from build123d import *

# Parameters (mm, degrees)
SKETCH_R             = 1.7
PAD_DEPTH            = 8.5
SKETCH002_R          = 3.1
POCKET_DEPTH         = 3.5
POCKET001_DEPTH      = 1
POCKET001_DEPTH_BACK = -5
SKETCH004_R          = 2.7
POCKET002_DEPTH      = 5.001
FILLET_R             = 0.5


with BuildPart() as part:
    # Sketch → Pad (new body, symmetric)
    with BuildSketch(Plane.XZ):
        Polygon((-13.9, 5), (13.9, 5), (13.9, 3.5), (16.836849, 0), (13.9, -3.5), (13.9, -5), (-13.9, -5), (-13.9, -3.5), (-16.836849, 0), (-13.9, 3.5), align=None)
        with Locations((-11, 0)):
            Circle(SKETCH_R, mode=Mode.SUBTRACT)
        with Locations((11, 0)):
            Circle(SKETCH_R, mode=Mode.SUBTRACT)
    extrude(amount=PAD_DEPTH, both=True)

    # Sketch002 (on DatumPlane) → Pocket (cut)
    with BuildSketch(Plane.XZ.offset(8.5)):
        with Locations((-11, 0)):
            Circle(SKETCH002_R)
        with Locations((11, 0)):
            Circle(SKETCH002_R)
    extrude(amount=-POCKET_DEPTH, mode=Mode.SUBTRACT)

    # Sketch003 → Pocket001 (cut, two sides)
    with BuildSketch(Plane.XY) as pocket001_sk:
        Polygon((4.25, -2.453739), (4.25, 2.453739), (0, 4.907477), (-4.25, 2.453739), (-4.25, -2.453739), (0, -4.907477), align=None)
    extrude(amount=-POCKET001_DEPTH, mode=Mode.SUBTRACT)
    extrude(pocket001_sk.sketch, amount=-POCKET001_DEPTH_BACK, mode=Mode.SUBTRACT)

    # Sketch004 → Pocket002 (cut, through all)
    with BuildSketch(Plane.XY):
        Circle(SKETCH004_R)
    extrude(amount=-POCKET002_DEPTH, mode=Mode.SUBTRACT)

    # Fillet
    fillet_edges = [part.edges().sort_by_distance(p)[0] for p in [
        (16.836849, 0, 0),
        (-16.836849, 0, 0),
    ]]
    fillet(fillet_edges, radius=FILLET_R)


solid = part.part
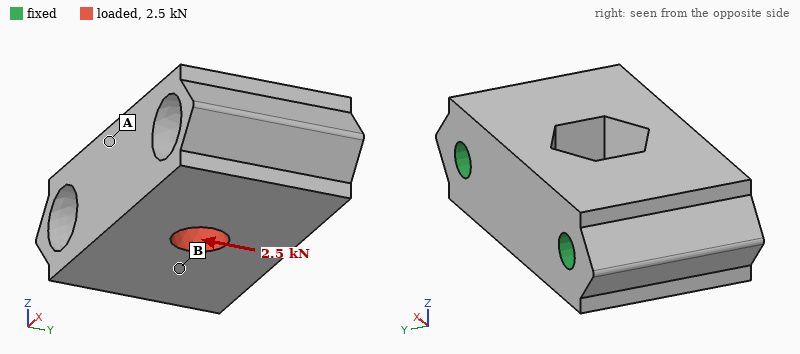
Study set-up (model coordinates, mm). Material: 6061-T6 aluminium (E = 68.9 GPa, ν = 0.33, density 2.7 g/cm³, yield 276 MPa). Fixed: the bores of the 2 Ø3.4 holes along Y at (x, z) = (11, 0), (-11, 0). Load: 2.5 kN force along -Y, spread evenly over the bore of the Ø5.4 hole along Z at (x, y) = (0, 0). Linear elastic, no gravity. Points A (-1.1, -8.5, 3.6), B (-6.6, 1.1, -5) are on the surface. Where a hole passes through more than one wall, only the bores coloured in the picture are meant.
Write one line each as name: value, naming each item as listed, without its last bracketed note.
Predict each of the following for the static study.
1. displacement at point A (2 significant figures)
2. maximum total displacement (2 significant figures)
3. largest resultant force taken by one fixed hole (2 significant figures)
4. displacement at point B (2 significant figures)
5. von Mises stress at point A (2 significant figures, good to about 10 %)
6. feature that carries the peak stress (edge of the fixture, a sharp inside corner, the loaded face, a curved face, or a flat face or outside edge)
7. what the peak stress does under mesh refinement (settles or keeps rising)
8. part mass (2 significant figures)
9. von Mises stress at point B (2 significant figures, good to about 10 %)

displacement at point A: 3.0 µm
maximum total displacement: 8.2 µm
largest resultant force taken by one fixed hole: 1.3 kN
displacement at point B: 2.8 µm
von Mises stress at point A: 14 MPa
feature that carries the peak stress: edge of the fixture
what the peak stress does under mesh refinement: keeps rising
part mass: 11 g
von Mises stress at point B: 27 MPa
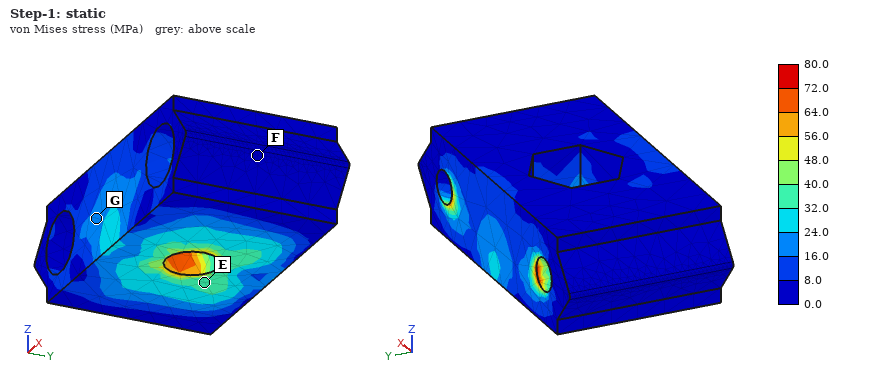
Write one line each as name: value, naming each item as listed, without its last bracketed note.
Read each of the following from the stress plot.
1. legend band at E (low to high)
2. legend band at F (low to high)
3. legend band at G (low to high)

legend band at E: 32.0 to 40.0 MPa
legend band at F: 0.0 to 8.0 MPa
legend band at G: 16.0 to 24.0 MPa
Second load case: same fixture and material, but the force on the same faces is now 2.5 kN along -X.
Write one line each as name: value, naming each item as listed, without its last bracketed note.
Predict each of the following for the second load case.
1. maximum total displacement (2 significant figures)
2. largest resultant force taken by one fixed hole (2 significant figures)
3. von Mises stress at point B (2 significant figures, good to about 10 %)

maximum total displacement: 3.9 µm
largest resultant force taken by one fixed hole: 1.3 kN
von Mises stress at point B: 25 MPa
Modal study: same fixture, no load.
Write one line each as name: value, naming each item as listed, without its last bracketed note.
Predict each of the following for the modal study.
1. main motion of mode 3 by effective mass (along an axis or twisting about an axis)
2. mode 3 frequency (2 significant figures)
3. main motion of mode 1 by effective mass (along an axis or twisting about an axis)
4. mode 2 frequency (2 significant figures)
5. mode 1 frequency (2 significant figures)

main motion of mode 3 by effective mass: along Y
mode 3 frequency: 65 kHz
main motion of mode 1 by effective mass: along Z
mode 2 frequency: 58 kHz
mode 1 frequency: 45 kHz
